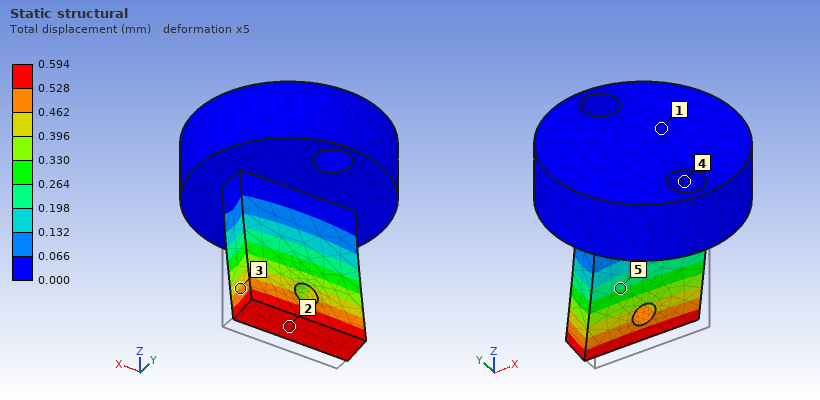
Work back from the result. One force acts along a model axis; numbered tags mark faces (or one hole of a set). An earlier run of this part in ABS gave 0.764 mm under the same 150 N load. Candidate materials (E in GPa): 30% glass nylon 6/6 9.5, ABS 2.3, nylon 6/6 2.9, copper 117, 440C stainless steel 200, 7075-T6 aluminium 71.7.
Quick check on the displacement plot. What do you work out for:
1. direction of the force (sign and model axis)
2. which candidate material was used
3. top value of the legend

+Y
nylon 6/6
0.594 mm
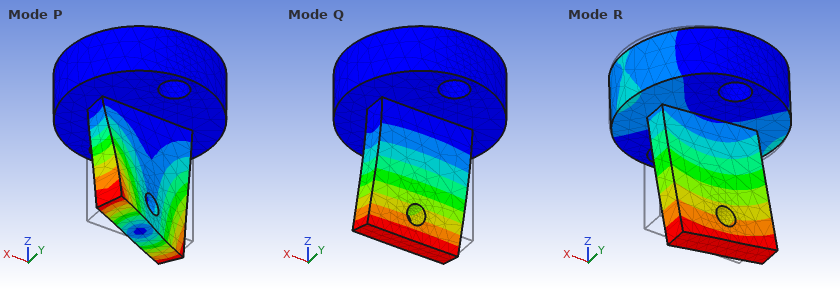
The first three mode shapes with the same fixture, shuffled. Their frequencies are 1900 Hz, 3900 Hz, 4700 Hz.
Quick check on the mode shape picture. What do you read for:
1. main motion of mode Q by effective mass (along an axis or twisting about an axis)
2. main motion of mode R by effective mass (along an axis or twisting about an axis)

along Y
along X
